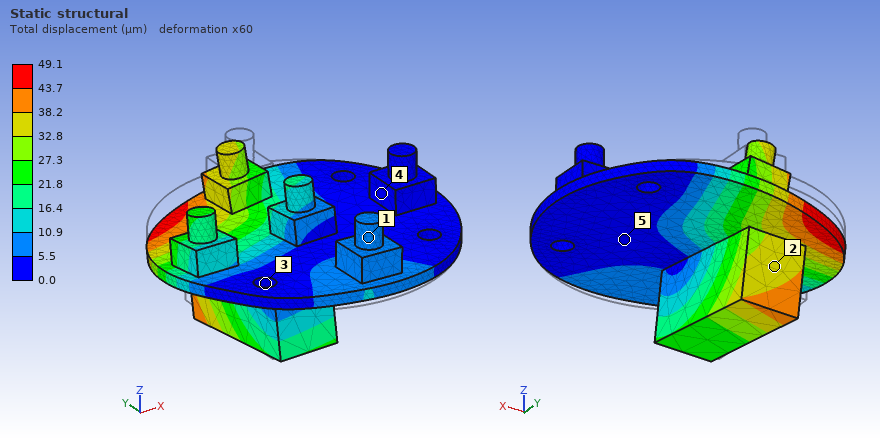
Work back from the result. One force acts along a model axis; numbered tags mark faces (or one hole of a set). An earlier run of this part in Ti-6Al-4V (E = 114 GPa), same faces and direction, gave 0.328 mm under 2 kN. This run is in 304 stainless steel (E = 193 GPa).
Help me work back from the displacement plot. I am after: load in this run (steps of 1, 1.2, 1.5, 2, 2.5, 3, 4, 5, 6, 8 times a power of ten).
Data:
500 N
